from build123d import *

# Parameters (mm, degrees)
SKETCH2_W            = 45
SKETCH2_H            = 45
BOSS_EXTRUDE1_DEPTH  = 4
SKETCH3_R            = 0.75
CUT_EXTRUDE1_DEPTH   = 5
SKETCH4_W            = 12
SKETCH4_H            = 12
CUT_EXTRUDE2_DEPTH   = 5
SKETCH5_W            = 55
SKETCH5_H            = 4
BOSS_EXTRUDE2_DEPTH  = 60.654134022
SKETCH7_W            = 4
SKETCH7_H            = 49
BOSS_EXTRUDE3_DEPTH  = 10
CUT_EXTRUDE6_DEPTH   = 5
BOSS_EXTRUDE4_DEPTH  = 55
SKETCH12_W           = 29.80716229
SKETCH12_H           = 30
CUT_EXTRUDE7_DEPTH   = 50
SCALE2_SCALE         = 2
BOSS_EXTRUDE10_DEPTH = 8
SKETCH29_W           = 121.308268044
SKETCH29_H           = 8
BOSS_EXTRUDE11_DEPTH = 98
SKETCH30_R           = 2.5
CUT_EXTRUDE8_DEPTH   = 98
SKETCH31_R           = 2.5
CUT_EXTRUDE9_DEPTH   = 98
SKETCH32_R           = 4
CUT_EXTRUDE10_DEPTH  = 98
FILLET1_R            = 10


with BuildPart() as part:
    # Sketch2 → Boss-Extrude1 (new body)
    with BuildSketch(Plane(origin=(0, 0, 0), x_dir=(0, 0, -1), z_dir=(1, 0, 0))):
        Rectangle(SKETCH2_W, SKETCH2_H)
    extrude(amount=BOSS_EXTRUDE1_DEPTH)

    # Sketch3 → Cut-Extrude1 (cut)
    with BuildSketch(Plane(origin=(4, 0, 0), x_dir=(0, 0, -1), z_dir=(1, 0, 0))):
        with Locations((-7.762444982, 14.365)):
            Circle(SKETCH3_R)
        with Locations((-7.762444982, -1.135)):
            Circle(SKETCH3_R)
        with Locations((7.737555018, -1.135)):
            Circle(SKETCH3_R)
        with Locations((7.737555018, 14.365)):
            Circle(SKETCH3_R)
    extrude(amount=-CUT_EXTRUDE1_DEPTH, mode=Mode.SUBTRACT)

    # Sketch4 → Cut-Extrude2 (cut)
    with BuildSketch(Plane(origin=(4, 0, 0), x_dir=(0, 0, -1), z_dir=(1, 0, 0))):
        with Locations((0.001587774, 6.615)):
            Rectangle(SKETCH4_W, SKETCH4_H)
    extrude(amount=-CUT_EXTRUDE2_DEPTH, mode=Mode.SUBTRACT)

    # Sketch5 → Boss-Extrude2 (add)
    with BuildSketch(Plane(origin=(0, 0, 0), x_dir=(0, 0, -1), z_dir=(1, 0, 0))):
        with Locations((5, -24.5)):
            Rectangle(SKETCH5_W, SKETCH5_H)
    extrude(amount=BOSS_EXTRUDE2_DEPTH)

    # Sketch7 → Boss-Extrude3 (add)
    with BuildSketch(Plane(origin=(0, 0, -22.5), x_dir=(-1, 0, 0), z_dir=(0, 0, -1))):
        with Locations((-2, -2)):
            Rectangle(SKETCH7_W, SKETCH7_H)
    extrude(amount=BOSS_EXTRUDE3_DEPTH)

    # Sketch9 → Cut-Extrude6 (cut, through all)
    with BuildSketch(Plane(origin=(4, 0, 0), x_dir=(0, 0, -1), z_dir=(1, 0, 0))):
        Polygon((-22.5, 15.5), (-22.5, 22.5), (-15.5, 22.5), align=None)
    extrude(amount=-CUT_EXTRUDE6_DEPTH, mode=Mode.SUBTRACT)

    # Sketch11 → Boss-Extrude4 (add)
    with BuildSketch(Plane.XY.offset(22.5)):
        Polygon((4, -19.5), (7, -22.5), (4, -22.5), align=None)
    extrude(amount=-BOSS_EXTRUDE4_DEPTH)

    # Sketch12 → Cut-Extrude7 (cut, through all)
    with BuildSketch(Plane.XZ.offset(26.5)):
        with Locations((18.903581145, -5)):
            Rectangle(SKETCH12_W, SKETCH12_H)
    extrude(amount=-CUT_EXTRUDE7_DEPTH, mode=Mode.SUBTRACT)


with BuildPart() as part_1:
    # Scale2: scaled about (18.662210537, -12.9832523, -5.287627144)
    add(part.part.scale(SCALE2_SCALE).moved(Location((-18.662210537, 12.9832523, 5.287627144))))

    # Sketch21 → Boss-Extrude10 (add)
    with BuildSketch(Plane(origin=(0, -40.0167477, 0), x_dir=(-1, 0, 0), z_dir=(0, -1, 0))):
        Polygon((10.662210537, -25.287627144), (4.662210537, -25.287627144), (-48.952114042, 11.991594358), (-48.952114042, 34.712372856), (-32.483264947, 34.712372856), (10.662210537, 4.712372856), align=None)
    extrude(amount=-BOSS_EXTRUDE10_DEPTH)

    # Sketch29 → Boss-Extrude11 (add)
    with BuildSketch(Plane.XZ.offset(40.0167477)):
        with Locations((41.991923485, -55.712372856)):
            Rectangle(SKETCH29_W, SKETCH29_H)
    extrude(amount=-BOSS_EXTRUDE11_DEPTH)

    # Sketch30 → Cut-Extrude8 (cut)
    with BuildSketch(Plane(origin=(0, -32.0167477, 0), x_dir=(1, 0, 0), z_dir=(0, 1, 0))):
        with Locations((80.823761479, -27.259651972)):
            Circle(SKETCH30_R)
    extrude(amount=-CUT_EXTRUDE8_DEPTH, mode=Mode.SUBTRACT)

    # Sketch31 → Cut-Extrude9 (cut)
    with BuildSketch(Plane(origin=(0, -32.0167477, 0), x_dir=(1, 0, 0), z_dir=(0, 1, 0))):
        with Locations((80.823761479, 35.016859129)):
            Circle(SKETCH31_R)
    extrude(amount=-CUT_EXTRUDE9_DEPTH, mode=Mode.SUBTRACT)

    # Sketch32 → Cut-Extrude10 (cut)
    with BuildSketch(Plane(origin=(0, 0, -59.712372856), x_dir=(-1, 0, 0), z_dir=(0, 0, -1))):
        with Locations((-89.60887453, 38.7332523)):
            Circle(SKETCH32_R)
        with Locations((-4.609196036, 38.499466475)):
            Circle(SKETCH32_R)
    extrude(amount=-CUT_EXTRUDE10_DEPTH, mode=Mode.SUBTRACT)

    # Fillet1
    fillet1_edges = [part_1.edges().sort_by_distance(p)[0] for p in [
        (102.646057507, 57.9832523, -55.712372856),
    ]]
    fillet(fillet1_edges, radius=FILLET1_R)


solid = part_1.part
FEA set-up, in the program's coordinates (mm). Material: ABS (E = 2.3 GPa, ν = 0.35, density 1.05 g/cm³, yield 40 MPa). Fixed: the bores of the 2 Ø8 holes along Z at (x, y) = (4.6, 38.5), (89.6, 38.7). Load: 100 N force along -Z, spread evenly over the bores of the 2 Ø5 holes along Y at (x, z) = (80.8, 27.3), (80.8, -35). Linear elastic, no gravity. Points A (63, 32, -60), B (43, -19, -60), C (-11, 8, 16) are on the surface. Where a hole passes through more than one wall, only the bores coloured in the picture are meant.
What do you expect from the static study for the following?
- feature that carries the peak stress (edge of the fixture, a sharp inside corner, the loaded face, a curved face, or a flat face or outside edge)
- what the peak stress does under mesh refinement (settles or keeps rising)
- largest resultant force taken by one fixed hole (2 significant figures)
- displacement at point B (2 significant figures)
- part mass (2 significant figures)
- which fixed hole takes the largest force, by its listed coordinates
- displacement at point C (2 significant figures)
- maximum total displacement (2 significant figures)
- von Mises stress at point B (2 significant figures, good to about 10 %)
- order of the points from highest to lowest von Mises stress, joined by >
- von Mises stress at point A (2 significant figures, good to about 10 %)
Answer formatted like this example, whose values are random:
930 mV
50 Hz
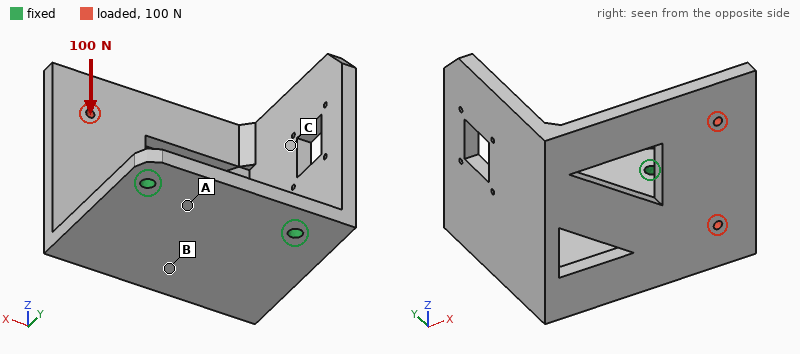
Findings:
edge of the fixture
keeps rising
79 N
0.63 mm
260 g
(89.6, 38.7)
0.71 mm
2.0 mm
1.5 MPa
A > B > C
2.2 MPa
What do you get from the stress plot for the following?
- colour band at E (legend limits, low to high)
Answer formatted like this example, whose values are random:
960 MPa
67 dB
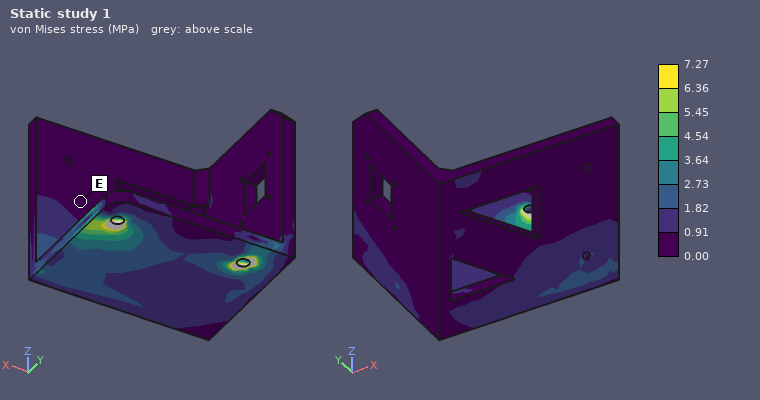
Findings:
0.00 to 0.91 MPa
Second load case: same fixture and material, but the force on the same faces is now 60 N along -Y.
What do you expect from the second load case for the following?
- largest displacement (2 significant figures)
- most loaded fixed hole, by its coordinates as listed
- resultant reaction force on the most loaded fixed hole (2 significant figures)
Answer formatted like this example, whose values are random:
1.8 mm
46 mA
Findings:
1.7 mm
(89.6, 38.7)
55 N
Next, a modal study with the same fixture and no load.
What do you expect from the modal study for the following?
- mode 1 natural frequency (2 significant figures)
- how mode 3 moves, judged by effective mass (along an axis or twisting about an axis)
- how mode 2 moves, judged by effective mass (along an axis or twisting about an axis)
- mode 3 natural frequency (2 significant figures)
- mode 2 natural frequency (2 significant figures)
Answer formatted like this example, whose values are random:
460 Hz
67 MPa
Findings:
110 Hz
along Z
along X
260 Hz
140 Hz
